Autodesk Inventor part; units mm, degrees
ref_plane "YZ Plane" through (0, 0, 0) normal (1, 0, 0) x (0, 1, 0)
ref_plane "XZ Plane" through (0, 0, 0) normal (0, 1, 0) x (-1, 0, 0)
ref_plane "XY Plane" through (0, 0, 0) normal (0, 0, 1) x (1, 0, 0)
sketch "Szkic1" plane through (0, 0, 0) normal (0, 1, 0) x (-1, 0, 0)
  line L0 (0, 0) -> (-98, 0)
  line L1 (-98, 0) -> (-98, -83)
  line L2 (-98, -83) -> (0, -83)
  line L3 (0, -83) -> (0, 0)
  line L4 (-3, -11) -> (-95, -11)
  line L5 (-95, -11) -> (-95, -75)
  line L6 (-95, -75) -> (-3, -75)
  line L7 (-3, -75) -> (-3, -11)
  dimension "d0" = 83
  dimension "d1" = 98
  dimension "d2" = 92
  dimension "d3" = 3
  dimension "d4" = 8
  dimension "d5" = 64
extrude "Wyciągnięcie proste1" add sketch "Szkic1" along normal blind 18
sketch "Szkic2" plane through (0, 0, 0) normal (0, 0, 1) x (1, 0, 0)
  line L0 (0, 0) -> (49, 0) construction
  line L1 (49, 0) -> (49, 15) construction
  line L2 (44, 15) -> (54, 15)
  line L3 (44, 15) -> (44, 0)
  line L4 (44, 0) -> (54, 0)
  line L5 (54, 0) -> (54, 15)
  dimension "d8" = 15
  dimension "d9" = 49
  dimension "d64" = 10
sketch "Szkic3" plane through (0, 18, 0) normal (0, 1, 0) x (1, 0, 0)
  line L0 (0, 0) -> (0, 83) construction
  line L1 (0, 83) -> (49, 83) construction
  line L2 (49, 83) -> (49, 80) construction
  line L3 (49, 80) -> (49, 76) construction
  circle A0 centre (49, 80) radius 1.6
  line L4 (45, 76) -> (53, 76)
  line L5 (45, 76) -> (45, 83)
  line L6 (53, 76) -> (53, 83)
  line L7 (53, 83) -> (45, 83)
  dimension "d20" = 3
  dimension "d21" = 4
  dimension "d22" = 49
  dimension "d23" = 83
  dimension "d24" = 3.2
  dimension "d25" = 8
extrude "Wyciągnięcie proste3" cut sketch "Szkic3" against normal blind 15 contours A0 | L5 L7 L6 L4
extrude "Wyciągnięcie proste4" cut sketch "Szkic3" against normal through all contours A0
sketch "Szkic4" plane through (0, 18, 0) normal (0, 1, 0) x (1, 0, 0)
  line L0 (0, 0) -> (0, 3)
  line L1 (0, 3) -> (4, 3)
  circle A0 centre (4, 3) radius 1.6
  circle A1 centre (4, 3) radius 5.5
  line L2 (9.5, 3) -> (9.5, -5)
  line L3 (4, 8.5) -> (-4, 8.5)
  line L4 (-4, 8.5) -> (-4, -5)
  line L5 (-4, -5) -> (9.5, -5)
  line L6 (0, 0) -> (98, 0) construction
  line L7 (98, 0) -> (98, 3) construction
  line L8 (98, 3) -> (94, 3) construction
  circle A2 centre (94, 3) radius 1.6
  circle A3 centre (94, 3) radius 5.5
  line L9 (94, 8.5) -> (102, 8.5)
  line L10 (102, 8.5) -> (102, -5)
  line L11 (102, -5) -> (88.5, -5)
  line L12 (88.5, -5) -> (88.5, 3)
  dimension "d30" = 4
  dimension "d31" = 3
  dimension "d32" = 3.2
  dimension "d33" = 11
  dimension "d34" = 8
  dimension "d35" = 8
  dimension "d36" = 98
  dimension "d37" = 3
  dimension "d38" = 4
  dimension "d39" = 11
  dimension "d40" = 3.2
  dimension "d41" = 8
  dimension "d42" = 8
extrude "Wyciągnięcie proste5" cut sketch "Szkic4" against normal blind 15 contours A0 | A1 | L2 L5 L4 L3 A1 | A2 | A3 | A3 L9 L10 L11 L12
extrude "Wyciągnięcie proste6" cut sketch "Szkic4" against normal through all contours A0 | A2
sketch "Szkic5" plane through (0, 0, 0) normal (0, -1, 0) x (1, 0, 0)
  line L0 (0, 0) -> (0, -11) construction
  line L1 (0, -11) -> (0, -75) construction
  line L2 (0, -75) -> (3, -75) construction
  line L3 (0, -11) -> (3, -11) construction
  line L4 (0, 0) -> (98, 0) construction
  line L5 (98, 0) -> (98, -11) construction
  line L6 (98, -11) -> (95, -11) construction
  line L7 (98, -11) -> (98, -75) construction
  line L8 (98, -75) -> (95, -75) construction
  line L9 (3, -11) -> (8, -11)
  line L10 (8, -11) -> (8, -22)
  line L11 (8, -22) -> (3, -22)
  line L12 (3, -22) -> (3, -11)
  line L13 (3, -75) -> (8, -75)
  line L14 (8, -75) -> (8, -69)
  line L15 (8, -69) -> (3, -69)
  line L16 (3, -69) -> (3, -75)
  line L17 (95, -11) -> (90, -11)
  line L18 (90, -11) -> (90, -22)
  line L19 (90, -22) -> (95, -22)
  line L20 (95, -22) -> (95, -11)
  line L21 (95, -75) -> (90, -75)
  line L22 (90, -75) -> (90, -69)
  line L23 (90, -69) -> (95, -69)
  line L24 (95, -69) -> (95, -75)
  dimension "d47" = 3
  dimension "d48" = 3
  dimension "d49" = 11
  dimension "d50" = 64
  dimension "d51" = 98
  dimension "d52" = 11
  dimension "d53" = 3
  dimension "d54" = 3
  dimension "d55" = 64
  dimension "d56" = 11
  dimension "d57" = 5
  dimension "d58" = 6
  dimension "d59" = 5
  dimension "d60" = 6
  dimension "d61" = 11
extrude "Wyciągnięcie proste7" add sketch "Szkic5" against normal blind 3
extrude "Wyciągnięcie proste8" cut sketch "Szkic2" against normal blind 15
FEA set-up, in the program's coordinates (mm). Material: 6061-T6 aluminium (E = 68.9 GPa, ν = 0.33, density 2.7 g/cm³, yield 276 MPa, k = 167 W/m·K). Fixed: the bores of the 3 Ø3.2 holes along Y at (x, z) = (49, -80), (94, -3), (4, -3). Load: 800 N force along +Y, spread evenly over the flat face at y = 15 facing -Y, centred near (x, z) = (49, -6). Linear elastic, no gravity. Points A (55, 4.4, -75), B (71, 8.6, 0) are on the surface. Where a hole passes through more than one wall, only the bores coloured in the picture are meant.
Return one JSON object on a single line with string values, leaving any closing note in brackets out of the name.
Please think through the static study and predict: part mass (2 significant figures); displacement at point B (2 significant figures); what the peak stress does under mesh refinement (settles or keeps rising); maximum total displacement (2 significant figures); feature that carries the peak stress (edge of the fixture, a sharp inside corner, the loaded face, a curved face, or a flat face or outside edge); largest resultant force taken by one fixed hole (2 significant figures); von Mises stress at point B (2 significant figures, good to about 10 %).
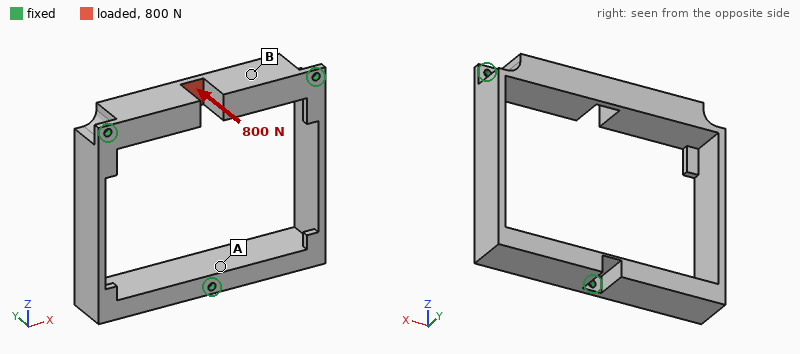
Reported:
{"part mass": "98 g", "displacement at point B": "25 µm", "what the peak stress does under mesh refinement": "keeps rising", "maximum total displacement": "47 µm", "feature that carries the peak stress": "edge of the fixture", "largest resultant force taken by one fixed hole": "1.1 kN", "von Mises stress at point B": "9.3 MPa"}
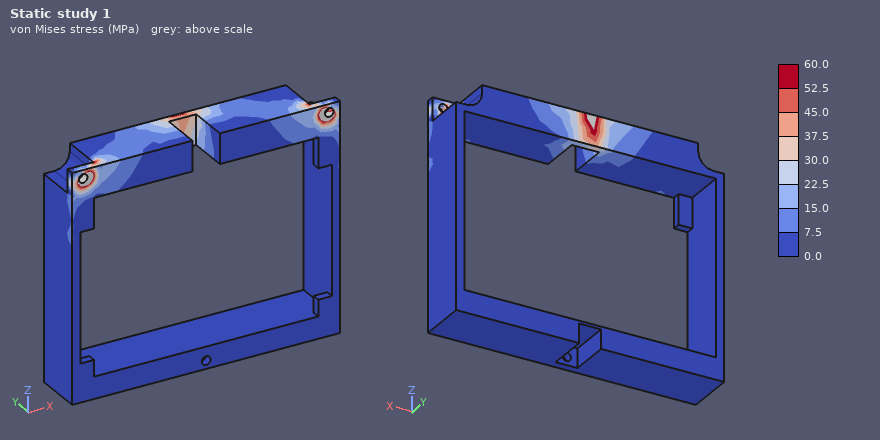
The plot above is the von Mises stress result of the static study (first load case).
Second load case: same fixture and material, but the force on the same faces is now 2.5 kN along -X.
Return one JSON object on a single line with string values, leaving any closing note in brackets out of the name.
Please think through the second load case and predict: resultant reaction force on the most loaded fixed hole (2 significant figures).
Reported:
{"resultant reaction force on the most loaded fixed hole": "1.3 kN"}
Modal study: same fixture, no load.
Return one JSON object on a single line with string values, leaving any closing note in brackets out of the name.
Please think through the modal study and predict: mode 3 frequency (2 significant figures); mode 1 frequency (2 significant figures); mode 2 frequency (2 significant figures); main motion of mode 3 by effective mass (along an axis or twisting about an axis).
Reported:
{"mode 3 frequency": "3000 Hz", "mode 1 frequency": "1200 Hz", "mode 2 frequency": "2500 Hz", "main motion of mode 3 by effective mass": "along Y"}
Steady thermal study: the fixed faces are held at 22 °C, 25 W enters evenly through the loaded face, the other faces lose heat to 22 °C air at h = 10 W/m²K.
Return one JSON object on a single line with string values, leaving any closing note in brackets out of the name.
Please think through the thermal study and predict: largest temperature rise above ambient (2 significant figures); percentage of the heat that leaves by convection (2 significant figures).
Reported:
{"largest temperature rise above ambient": "38 K", "percentage of the heat that leaves by convection": "5.9 %"}
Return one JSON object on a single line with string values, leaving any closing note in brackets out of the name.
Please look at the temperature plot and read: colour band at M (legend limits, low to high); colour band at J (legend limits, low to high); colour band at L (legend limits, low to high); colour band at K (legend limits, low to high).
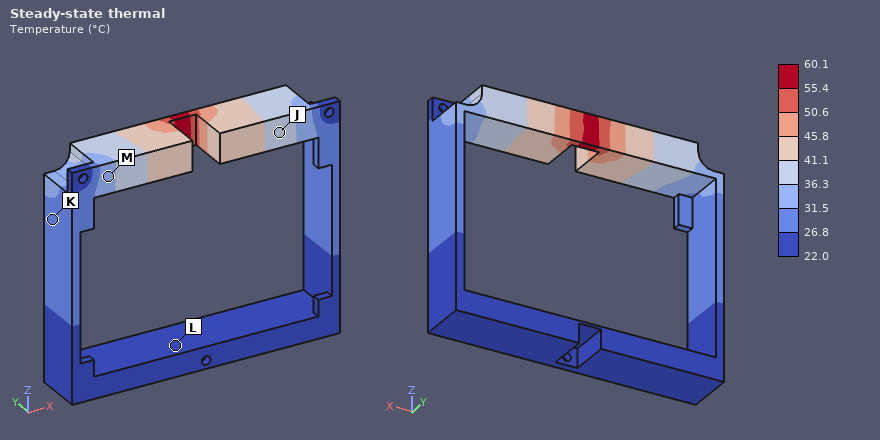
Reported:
{"colour band at M": "31.5 to 36.3 °C", "colour band at J": "36.3 to 41.1 °C", "colour band at L": "22.0 to 26.8 °C", "colour band at K": "26.8 to 31.5 °C"}
